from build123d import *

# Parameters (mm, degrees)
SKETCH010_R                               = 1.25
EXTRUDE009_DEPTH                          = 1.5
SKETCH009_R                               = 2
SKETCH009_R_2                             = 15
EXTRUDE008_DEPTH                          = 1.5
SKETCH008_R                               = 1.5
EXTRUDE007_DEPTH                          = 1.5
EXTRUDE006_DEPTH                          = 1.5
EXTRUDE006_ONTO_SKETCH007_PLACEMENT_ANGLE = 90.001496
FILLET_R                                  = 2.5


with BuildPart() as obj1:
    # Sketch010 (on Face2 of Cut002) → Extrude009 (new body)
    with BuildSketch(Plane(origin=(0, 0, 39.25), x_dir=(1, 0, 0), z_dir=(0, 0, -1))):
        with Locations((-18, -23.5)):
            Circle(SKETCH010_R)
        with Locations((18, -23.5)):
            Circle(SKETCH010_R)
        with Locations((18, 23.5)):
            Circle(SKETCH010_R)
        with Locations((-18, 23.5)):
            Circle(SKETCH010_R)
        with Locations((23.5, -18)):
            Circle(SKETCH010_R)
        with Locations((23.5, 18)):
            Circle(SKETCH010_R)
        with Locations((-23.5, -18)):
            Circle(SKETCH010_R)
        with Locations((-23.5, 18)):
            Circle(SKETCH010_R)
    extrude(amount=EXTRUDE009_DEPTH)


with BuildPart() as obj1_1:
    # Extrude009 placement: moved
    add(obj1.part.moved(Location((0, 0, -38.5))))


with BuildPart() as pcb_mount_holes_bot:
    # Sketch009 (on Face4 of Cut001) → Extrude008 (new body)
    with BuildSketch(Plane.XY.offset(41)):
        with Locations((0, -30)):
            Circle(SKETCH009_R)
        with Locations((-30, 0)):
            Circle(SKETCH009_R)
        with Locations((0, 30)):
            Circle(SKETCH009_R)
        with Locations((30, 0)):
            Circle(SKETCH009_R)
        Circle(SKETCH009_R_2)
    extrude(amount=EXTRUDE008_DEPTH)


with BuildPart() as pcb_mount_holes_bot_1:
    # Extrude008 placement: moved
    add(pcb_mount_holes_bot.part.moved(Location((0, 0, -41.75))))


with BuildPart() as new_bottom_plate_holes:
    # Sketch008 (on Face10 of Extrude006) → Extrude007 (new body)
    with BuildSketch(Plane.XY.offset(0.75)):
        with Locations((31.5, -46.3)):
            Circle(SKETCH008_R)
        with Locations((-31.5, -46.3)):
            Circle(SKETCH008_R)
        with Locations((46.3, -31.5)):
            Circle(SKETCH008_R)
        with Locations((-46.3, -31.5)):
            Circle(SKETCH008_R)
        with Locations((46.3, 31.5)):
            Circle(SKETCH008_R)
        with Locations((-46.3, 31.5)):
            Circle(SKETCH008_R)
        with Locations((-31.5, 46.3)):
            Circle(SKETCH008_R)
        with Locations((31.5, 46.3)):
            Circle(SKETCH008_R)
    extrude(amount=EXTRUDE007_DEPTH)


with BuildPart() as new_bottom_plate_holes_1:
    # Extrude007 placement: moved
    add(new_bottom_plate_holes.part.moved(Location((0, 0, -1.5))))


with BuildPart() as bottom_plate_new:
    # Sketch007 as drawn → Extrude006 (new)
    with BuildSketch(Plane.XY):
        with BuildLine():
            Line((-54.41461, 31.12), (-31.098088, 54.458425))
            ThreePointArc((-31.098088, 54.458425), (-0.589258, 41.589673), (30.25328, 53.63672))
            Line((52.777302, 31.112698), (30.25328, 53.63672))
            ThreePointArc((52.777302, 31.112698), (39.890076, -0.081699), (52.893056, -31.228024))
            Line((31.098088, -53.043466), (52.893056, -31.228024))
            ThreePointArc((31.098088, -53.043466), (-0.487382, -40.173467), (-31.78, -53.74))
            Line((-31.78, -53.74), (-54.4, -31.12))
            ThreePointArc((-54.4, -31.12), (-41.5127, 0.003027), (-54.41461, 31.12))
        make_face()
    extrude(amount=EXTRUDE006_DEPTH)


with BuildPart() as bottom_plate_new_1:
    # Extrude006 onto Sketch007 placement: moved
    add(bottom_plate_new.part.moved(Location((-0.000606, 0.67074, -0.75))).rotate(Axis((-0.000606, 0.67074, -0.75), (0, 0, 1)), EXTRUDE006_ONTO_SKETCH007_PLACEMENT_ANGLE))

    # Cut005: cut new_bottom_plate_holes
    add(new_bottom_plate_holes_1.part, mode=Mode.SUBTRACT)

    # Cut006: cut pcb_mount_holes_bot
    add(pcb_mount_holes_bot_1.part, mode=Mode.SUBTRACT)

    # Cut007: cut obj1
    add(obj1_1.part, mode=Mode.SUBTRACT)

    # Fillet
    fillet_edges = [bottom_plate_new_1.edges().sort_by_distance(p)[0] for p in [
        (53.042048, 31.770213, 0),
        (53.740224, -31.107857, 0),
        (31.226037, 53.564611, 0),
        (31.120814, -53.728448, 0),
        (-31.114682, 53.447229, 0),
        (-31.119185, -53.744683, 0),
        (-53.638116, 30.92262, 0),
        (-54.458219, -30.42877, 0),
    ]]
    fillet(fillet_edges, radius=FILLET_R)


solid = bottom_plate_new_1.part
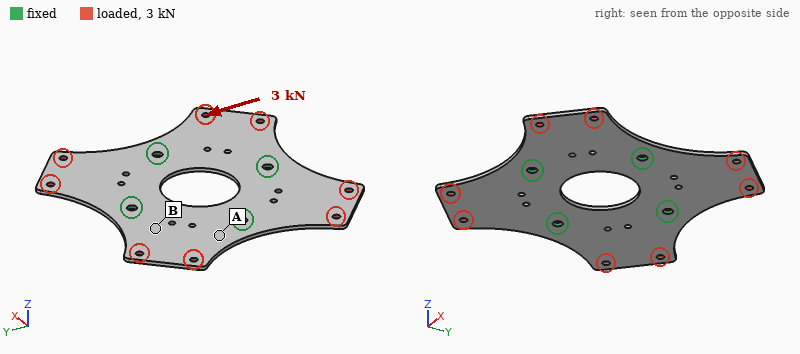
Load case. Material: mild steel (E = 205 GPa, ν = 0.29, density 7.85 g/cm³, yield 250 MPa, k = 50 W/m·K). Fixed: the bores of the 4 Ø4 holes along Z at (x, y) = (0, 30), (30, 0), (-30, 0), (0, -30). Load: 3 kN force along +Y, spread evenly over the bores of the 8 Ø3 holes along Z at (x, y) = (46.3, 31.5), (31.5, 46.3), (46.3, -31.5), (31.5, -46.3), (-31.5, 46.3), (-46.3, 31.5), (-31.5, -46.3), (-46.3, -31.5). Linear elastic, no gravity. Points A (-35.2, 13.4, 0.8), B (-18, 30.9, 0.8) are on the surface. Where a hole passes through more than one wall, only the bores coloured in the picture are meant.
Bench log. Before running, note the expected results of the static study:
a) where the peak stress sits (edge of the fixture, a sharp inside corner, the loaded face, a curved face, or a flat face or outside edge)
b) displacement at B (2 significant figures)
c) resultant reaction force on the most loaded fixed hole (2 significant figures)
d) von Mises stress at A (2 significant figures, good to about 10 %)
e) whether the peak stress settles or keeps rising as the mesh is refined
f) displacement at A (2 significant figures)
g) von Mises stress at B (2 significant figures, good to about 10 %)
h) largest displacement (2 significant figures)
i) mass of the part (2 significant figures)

edge of the fixture
1.9 µm
1.3 kN
27 MPa
keeps rising
2.7 µm
10 MPa
8.3 µm
88 g
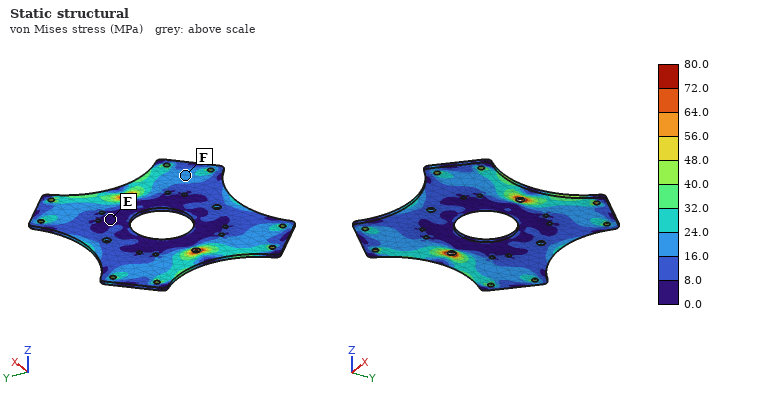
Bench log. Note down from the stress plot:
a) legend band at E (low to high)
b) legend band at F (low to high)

0.0 to 8.0 MPa
16.0 to 24.0 MPa
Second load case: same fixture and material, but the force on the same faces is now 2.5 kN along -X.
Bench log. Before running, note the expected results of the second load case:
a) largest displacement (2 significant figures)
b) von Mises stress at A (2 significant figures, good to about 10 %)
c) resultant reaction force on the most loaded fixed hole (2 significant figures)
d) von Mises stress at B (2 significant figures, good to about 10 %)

6.7 µm
8.3 MPa
1.1 kN
16 MPa
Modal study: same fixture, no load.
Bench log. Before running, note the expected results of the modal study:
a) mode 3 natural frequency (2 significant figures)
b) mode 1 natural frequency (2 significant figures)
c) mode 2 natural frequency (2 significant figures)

930 Hz
910 Hz
930 Hz
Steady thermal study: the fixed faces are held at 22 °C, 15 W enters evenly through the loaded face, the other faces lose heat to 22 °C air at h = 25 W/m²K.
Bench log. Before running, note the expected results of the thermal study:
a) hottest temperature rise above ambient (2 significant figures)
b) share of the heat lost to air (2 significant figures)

42 K
43 %
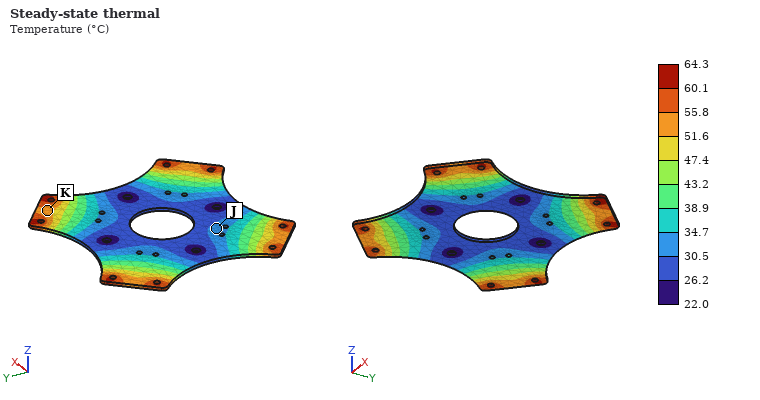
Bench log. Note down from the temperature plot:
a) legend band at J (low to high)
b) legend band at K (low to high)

30.5 to 34.7 °C
51.6 to 55.8 °C
